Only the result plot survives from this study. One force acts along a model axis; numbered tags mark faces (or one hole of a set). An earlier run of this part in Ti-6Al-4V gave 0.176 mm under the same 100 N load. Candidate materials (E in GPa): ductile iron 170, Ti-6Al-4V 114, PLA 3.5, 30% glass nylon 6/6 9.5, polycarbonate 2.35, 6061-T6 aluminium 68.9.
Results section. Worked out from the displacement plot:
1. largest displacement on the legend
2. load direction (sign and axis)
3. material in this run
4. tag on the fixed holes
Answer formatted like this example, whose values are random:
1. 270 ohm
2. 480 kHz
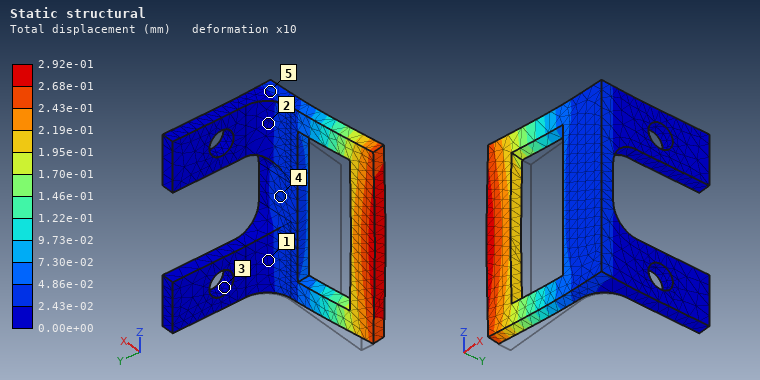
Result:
1. 2.92e-01 mm
2. -Y
3. 6061-T6 aluminium
4. 3
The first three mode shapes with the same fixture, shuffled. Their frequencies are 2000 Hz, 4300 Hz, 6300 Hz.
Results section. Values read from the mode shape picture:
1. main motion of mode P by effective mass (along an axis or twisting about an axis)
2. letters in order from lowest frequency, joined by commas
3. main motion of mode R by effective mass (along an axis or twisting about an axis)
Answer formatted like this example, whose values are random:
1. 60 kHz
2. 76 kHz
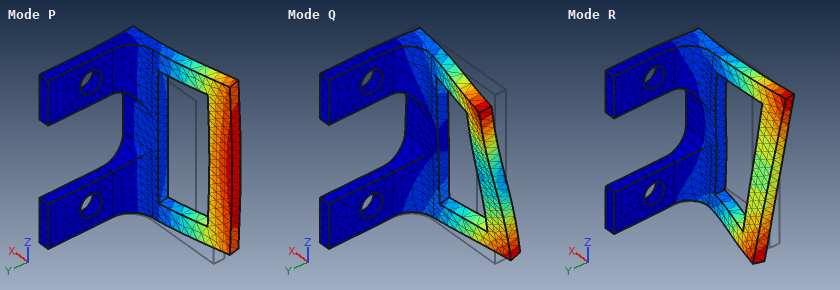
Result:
1. along Y
2. P, Q, R
3. along Z
